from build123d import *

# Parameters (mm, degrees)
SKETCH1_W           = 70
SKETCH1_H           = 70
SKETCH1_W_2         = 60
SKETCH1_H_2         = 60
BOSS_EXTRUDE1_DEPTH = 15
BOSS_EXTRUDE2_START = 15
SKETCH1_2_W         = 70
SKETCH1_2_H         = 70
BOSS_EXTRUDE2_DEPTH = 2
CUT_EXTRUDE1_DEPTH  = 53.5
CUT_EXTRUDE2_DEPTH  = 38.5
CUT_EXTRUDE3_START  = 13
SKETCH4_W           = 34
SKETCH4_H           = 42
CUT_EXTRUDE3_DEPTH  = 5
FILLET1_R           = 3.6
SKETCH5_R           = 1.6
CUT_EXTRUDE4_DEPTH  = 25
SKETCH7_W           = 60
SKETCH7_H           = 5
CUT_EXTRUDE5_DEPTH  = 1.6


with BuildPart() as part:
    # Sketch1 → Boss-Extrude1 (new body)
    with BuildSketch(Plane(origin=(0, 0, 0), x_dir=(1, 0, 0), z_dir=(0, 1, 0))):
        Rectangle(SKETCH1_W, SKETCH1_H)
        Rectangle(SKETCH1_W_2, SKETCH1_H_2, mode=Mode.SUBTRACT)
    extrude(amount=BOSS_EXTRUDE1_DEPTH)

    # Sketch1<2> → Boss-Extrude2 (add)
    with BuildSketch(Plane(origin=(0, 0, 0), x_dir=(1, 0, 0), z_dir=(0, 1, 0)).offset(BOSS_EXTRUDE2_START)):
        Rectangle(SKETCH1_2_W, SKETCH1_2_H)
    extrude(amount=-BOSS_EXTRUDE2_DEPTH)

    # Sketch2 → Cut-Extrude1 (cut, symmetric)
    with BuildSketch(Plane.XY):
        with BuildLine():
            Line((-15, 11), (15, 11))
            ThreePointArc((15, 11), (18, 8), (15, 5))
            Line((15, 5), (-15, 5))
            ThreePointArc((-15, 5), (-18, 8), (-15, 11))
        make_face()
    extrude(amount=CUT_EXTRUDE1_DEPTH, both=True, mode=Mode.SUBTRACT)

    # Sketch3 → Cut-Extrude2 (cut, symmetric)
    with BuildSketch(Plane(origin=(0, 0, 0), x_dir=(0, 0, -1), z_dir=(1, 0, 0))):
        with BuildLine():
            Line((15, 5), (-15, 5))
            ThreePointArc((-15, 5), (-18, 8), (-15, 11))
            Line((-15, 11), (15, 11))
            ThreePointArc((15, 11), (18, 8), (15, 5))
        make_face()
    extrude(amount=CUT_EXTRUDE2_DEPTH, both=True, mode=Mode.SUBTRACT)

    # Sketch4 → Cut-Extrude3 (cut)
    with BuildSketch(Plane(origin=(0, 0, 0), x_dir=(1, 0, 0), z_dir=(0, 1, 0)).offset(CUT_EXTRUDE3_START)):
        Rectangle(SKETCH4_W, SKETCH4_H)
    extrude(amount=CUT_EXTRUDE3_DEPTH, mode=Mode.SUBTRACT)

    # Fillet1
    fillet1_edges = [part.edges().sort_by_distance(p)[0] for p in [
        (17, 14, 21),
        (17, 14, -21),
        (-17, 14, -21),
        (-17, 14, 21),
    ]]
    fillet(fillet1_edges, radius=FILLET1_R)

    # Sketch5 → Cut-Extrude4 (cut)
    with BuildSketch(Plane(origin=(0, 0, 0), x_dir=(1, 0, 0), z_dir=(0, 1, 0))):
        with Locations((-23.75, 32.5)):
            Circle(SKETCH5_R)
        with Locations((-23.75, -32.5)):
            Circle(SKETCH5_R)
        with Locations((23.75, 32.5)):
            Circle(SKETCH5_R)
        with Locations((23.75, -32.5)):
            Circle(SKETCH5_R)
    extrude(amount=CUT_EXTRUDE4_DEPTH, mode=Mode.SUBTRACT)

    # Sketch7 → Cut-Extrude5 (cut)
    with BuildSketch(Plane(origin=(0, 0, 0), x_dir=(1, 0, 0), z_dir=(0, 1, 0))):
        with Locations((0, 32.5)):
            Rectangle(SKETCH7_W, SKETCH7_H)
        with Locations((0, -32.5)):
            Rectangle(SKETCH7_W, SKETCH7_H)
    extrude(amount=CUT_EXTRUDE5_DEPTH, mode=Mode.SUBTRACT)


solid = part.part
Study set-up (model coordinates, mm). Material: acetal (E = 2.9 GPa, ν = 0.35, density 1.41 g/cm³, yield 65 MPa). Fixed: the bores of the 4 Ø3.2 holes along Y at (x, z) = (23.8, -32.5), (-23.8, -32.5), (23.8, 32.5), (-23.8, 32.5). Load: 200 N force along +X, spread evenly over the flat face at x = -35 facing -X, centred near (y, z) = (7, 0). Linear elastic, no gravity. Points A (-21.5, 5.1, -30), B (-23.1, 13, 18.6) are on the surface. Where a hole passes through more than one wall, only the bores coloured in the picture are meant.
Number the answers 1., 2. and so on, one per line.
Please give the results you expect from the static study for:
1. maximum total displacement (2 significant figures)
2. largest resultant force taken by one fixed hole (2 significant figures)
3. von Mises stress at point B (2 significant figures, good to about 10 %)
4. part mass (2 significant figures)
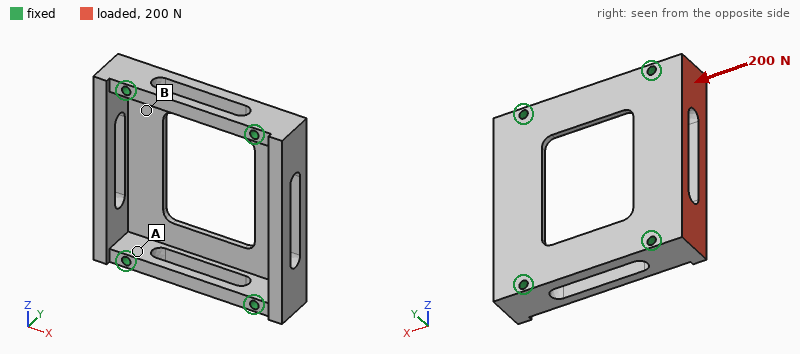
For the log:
1. 0.25 mm
2. 97 N
3. 3.4 MPa
4. 26 g
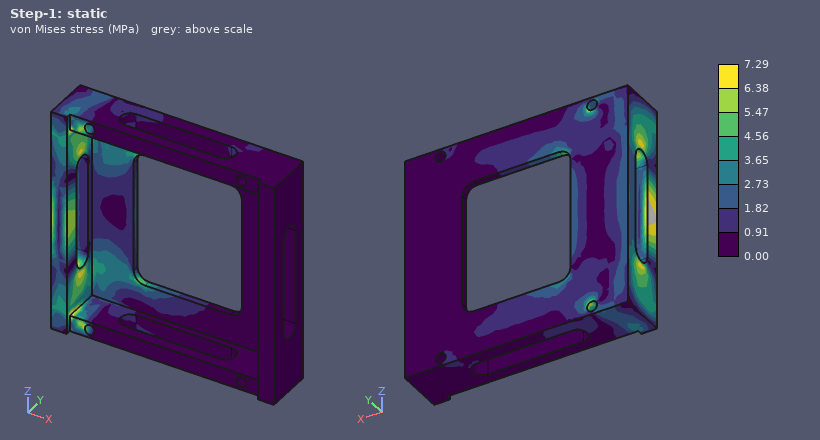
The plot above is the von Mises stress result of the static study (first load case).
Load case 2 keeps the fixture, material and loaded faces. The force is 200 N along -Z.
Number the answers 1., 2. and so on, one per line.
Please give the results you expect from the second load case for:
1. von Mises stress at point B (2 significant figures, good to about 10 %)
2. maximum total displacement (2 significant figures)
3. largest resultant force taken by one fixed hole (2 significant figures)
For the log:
1. 1.0 MPa
2. 42 µm
3. 100 N
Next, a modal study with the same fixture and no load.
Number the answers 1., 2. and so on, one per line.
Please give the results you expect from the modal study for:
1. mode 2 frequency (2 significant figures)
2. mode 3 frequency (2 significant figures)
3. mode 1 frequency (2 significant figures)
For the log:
1. 1800 Hz
2. 2300 Hz
3. 1700 Hz
